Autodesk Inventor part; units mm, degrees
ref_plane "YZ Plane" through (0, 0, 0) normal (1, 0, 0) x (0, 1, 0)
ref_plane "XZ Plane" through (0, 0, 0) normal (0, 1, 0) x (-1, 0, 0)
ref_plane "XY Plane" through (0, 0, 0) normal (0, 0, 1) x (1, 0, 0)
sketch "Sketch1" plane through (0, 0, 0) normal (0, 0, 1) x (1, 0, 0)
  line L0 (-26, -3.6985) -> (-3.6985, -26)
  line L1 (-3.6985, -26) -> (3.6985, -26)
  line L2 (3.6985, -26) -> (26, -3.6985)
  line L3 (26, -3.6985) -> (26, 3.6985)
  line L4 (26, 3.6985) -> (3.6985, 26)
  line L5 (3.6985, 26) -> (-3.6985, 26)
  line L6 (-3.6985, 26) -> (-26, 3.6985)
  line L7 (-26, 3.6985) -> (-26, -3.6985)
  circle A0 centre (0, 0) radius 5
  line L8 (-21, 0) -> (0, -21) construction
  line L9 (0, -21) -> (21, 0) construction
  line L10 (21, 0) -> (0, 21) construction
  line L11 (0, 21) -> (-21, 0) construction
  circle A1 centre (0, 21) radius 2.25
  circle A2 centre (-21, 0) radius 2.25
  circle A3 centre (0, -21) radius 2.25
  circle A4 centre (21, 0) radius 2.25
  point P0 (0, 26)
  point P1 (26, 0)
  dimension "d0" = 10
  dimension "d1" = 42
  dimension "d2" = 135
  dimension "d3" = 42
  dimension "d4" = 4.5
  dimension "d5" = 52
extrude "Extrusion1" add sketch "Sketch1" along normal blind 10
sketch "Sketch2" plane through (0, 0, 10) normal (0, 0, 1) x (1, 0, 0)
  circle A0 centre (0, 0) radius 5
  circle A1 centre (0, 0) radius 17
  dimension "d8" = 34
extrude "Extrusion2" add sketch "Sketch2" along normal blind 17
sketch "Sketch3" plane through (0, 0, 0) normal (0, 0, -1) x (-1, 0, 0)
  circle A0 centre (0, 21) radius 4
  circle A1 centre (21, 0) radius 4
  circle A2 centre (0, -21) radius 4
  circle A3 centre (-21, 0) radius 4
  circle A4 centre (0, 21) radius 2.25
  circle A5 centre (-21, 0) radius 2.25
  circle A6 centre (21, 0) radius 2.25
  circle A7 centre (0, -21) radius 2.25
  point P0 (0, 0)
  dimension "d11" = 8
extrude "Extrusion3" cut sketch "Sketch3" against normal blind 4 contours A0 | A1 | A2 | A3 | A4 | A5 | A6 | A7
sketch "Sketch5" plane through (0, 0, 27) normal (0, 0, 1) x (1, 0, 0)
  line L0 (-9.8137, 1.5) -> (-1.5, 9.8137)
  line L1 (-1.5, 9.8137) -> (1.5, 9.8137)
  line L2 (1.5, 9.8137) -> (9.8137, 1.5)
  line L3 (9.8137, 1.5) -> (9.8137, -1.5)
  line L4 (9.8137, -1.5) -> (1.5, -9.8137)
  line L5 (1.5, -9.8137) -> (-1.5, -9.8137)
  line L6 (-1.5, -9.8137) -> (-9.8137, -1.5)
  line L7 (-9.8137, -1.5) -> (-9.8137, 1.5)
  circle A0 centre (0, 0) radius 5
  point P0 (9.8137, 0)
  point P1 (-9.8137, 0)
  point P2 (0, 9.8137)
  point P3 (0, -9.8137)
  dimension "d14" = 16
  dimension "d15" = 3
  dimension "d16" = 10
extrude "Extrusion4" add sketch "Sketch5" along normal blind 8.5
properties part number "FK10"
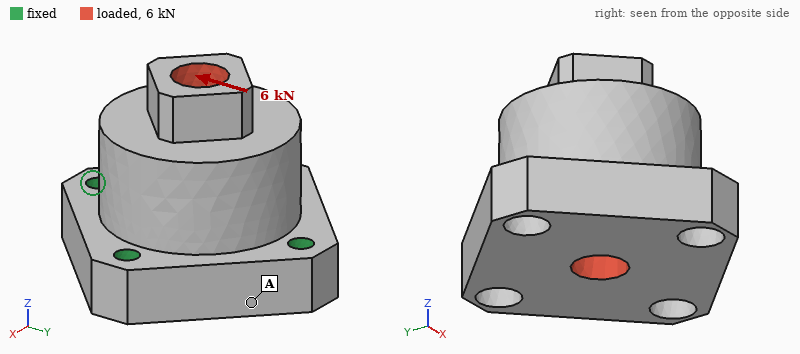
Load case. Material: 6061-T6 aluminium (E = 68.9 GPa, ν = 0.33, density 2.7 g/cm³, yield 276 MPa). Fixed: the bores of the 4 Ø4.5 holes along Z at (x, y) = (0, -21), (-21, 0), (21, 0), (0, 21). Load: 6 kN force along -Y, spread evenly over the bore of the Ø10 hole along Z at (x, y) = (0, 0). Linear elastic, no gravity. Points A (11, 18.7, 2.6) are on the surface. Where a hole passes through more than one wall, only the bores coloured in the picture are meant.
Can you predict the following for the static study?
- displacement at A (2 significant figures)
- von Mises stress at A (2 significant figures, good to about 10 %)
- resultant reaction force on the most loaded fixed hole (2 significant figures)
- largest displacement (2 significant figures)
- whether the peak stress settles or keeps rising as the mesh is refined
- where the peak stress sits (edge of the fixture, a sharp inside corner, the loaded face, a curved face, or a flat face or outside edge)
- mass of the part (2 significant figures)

4.0 µm
12 MPa
2.5 kN
19 µm
keeps rising
edge of the fixture
83 g
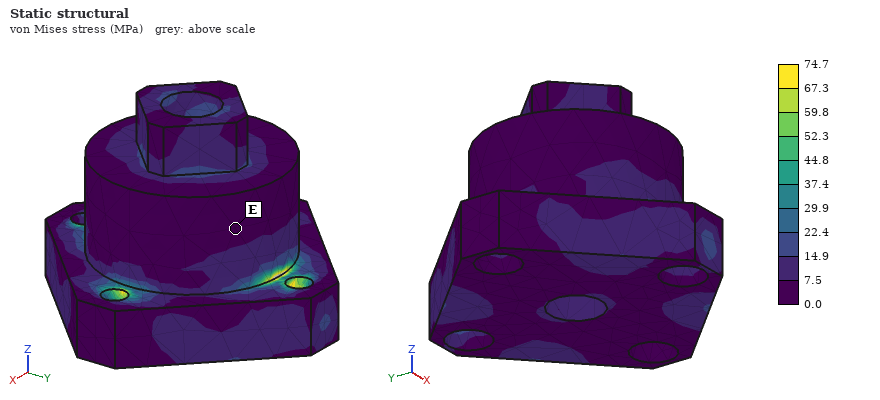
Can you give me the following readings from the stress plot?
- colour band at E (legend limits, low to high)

0.0 to 7.5 MPa
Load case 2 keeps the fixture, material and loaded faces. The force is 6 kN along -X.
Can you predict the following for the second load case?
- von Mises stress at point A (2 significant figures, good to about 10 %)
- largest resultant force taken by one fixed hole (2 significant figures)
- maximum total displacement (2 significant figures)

9.3 MPa
2.5 kN
19 µm
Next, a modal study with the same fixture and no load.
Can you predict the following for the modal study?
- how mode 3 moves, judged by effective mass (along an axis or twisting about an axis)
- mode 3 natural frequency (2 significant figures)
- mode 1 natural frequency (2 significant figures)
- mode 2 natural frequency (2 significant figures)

along Z
21 kHz
17 kHz
17 kHz
